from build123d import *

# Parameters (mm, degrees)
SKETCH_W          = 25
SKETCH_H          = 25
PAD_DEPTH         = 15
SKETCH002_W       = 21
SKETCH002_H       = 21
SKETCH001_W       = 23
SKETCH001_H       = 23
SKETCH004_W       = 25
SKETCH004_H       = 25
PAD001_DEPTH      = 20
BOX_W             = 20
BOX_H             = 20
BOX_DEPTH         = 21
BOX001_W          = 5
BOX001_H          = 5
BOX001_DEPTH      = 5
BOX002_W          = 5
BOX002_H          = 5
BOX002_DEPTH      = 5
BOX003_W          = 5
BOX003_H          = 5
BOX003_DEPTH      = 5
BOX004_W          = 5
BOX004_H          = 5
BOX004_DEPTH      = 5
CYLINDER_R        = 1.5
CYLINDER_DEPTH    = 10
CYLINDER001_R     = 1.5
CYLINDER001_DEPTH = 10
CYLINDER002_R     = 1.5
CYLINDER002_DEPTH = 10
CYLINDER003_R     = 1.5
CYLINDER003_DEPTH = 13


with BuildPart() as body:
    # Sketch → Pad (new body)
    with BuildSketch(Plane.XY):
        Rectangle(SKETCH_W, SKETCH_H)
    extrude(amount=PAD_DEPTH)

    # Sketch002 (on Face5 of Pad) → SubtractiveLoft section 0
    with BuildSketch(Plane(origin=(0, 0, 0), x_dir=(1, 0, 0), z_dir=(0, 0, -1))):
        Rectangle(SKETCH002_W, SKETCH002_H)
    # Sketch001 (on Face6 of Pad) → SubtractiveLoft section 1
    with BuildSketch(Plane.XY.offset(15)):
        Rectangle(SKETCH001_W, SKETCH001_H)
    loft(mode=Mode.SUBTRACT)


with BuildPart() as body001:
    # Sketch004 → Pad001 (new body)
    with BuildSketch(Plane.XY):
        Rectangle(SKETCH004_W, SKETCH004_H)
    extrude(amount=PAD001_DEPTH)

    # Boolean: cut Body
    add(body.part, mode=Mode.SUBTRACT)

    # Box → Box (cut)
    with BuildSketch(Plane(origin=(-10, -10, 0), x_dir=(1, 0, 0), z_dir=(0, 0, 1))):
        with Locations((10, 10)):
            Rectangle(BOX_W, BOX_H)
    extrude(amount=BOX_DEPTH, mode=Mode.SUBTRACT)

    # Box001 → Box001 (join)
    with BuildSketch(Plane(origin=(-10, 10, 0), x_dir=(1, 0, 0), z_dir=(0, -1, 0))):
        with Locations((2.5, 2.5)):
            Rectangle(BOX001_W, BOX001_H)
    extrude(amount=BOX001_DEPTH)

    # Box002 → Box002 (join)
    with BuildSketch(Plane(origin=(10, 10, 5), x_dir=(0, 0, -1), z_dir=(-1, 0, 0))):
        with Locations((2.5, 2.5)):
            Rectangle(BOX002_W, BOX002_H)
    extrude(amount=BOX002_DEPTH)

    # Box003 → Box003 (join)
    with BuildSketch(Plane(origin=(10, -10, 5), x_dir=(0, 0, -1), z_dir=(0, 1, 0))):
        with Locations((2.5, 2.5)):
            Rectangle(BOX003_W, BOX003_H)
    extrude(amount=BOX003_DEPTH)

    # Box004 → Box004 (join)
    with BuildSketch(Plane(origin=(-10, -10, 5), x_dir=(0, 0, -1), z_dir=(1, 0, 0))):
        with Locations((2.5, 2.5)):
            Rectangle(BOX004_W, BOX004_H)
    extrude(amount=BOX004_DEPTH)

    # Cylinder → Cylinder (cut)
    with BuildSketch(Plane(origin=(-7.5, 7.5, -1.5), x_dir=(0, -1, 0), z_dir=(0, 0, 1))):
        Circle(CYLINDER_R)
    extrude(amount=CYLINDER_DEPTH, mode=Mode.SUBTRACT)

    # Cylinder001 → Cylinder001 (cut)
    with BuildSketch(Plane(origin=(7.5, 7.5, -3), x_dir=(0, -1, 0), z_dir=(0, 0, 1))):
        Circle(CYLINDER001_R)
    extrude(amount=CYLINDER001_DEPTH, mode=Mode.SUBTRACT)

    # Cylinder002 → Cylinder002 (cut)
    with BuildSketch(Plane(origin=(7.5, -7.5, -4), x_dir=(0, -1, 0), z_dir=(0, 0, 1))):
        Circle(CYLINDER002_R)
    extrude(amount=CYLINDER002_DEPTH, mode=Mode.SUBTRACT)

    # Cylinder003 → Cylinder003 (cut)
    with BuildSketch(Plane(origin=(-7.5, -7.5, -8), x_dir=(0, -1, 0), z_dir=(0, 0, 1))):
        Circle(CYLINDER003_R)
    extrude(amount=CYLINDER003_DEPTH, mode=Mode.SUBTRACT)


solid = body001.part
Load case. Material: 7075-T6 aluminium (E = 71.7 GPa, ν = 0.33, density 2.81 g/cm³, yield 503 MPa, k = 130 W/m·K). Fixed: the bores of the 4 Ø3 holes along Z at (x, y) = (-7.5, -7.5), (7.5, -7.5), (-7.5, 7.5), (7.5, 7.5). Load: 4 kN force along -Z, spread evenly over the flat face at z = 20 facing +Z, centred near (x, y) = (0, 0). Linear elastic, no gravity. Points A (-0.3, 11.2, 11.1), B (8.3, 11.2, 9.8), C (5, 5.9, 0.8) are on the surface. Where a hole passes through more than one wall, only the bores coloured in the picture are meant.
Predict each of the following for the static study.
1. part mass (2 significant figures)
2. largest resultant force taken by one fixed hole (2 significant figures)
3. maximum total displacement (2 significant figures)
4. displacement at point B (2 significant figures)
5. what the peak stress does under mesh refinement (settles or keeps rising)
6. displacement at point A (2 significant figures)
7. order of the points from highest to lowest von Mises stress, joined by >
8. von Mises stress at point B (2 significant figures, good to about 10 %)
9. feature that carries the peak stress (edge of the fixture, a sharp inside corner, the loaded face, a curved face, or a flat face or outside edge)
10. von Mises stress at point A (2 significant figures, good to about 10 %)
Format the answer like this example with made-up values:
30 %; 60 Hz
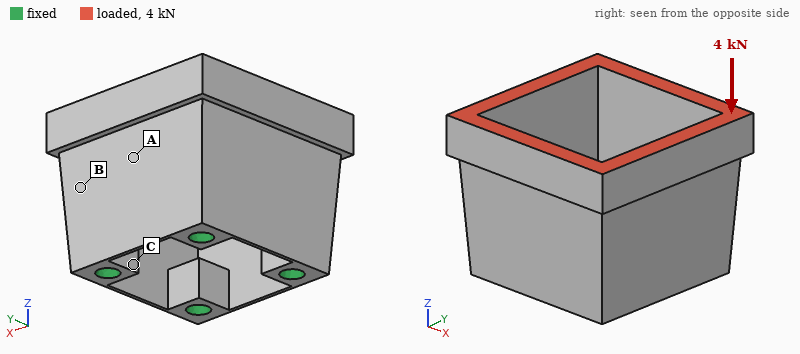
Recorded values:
7.7 g; 1.0 kN; 15 µm; 7.6 µm; keeps rising; 8.8 µm; B > A > C; 52 MPa; edge of the fixture; 33 MPa
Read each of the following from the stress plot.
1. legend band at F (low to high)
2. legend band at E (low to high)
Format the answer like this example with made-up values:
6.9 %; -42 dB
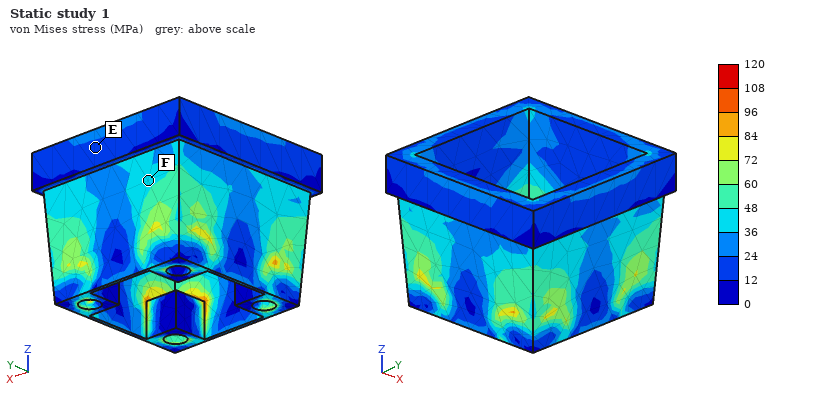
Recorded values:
36 to 48 MPa; 12 to 24 MPa
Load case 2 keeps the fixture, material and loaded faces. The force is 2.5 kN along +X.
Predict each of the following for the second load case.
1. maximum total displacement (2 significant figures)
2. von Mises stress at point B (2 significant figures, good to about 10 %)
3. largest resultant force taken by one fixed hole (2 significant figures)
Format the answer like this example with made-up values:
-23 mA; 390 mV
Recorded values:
0.14 mm; 66 MPa; 1.3 kN
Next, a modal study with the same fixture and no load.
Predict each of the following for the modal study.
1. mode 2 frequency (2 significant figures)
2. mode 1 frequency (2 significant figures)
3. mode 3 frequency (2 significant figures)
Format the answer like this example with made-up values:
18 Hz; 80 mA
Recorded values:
15 kHz; 12 kHz; 15 kHz
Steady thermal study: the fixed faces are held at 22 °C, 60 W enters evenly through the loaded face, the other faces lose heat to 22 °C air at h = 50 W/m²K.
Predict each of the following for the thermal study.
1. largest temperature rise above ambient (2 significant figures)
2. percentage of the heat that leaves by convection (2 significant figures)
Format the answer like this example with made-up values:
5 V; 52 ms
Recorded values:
70 K; 12 %
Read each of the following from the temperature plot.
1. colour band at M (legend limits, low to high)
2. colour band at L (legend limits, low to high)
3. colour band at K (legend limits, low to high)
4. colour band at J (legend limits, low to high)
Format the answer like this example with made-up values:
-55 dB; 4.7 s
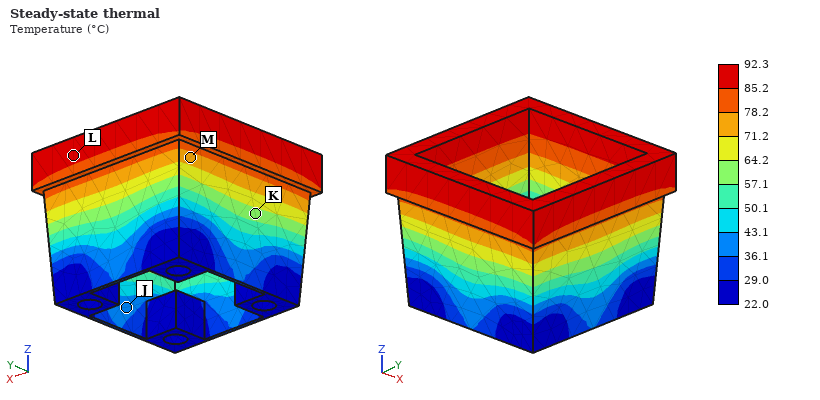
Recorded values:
71.2 to 78.2 °C; 85.2 to 92.3 °C; 57.1 to 64.2 °C; 36.1 to 43.1 °C
